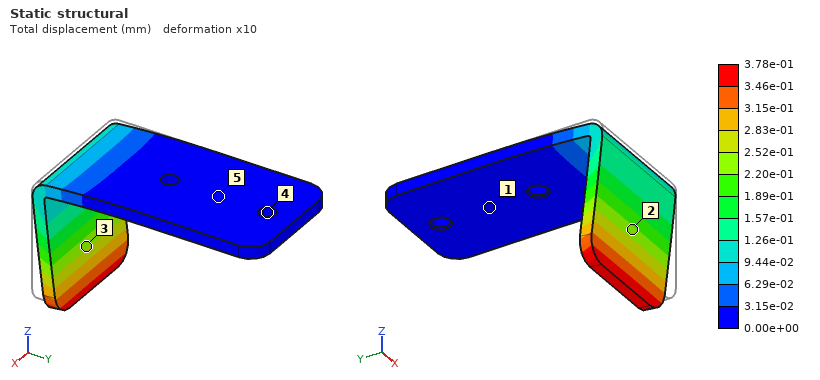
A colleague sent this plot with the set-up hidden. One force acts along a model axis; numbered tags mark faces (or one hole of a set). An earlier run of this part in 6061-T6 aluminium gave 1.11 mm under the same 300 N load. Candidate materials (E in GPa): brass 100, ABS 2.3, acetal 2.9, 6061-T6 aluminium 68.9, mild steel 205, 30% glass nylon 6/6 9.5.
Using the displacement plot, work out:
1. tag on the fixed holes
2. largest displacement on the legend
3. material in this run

4
3.78e-01 mm
mild steel
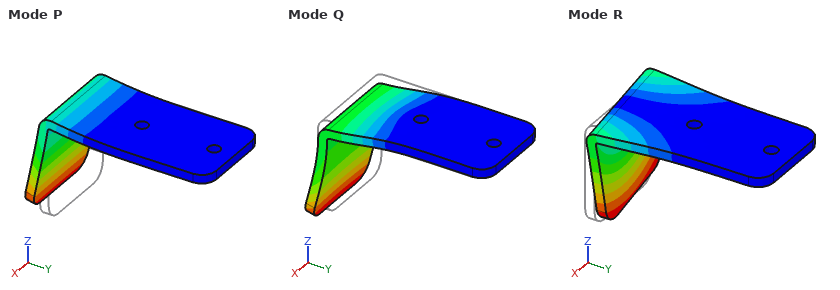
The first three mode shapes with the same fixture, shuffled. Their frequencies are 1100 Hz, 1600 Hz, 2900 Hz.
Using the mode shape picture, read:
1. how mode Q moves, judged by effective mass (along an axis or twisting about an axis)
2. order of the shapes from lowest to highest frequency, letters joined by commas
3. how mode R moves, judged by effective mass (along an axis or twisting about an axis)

along Z
P, R, Q
along X
